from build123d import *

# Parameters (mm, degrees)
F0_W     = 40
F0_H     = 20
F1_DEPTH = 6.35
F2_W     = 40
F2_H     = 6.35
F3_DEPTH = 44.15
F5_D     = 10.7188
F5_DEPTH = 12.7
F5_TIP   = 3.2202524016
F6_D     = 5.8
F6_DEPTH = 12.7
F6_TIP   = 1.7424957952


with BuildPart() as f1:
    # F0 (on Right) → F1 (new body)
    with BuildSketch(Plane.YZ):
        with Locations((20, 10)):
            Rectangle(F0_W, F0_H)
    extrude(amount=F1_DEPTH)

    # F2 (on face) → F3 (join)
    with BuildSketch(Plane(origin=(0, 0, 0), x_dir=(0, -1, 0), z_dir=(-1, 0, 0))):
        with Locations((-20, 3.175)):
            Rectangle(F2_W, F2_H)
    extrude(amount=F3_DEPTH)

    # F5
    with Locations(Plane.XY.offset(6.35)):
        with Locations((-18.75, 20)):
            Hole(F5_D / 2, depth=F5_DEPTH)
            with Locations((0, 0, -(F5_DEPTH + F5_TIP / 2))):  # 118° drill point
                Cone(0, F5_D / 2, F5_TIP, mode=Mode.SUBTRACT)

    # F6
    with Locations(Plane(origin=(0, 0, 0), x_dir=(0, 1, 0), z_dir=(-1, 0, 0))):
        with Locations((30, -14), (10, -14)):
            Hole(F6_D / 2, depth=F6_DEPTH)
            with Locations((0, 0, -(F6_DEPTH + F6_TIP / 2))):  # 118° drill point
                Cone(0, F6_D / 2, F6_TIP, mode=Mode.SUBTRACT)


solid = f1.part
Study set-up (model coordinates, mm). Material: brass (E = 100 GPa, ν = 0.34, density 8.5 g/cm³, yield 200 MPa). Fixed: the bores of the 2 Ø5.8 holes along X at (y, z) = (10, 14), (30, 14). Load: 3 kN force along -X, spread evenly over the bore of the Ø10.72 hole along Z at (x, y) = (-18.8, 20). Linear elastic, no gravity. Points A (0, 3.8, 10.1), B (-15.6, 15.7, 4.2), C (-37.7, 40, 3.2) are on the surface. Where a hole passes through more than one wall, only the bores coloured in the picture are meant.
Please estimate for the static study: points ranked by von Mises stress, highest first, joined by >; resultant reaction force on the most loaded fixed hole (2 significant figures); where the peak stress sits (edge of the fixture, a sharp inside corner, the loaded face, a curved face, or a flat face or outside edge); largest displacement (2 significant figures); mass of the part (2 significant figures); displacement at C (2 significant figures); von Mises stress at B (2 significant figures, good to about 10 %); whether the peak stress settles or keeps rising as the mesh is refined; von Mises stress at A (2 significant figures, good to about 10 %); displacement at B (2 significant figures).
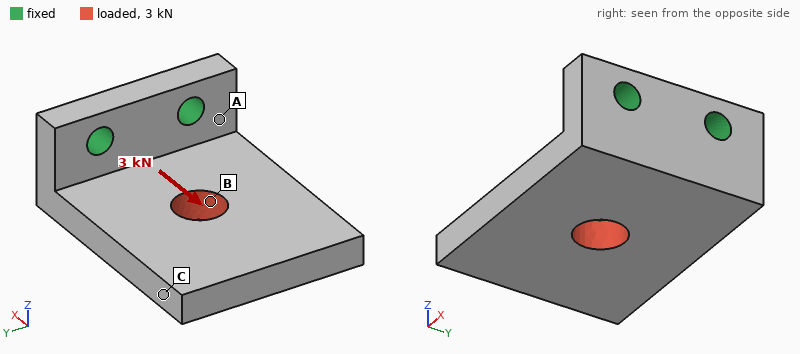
A > B > C
1.5 kN
edge of the fixture
93 µm
130 g
79 µm
24 MPa
keeps rising
47 MPa
39 µm
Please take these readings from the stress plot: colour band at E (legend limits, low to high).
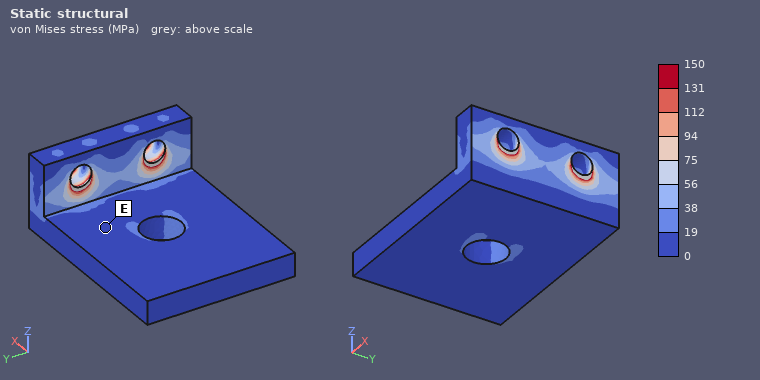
0 to 19 MPa
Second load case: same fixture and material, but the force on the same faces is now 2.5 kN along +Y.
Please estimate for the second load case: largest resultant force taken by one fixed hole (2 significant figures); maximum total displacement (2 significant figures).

2.6 kN
82 µm
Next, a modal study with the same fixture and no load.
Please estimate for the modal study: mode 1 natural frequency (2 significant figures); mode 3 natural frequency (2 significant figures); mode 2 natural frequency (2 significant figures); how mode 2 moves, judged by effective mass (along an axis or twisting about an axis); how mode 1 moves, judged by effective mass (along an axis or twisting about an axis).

1200 Hz
4000 Hz
3000 Hz
along Y
along Z
